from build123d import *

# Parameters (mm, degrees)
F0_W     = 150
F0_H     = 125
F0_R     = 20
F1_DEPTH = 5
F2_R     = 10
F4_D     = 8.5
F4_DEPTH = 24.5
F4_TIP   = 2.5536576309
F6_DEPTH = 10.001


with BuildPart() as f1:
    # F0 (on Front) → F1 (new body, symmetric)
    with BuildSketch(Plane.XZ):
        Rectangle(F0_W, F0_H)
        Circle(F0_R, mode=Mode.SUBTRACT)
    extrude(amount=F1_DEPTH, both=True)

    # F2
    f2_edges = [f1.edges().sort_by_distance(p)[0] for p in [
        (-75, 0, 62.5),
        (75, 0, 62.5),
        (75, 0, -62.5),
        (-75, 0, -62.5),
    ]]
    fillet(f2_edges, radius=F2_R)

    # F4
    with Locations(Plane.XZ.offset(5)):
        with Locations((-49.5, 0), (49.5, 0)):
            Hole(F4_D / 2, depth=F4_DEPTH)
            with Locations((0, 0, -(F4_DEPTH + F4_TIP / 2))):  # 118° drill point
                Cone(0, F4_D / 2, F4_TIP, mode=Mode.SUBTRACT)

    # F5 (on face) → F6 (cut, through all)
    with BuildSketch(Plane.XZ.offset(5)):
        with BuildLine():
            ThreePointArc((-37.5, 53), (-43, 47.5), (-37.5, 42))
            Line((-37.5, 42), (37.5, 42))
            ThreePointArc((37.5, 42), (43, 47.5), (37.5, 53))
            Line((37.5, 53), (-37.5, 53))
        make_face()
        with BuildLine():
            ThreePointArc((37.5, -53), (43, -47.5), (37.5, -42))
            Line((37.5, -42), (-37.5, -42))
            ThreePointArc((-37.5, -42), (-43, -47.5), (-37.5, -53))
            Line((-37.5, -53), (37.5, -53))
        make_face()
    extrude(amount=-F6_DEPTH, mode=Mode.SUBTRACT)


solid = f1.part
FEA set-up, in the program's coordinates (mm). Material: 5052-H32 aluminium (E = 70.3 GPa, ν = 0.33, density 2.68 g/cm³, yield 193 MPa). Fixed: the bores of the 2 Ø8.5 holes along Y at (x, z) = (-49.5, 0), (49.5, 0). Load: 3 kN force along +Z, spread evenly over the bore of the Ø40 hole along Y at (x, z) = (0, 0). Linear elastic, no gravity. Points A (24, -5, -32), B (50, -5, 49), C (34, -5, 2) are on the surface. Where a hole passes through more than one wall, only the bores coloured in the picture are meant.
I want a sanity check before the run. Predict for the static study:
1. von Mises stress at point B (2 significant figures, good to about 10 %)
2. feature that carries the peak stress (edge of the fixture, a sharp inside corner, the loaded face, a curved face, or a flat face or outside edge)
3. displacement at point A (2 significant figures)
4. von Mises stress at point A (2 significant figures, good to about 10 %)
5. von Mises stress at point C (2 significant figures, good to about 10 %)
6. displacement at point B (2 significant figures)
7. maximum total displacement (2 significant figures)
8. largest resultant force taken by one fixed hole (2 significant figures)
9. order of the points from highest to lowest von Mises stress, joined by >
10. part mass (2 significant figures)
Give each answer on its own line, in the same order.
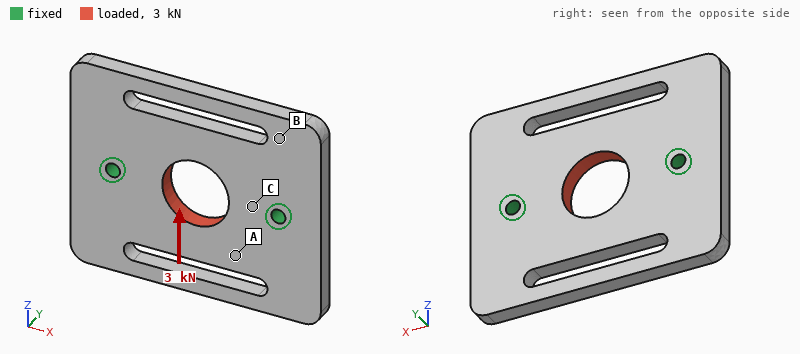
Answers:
1.4 MPa
edge of the fixture
2.9 µm
2.8 MPa
4.1 MPa
1.4 µm
4.7 µm
1.5 kN
C > A > B
410 g
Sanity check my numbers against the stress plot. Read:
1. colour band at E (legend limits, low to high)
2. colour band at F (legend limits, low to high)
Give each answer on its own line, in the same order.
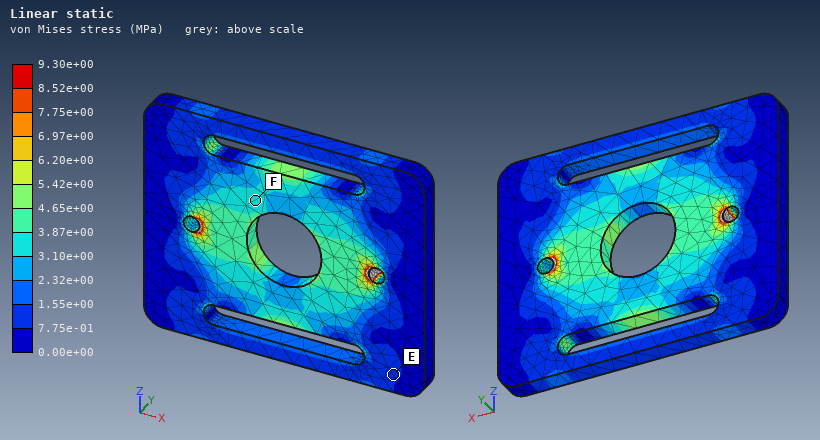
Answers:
7.75e-01 to 1.55e+00 MPa
3.10e+00 to 3.87e+00 MPa
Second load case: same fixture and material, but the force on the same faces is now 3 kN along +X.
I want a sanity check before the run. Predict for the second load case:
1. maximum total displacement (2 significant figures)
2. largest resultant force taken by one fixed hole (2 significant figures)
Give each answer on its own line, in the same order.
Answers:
2.7 µm
1.5 kN
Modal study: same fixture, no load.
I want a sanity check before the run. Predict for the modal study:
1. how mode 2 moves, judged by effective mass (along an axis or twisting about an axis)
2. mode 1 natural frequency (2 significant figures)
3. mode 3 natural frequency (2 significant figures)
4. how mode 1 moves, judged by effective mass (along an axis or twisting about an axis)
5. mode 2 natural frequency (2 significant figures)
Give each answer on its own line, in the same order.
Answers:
along Y
1600 Hz
2400 Hz
twisting about X
2000 Hz
